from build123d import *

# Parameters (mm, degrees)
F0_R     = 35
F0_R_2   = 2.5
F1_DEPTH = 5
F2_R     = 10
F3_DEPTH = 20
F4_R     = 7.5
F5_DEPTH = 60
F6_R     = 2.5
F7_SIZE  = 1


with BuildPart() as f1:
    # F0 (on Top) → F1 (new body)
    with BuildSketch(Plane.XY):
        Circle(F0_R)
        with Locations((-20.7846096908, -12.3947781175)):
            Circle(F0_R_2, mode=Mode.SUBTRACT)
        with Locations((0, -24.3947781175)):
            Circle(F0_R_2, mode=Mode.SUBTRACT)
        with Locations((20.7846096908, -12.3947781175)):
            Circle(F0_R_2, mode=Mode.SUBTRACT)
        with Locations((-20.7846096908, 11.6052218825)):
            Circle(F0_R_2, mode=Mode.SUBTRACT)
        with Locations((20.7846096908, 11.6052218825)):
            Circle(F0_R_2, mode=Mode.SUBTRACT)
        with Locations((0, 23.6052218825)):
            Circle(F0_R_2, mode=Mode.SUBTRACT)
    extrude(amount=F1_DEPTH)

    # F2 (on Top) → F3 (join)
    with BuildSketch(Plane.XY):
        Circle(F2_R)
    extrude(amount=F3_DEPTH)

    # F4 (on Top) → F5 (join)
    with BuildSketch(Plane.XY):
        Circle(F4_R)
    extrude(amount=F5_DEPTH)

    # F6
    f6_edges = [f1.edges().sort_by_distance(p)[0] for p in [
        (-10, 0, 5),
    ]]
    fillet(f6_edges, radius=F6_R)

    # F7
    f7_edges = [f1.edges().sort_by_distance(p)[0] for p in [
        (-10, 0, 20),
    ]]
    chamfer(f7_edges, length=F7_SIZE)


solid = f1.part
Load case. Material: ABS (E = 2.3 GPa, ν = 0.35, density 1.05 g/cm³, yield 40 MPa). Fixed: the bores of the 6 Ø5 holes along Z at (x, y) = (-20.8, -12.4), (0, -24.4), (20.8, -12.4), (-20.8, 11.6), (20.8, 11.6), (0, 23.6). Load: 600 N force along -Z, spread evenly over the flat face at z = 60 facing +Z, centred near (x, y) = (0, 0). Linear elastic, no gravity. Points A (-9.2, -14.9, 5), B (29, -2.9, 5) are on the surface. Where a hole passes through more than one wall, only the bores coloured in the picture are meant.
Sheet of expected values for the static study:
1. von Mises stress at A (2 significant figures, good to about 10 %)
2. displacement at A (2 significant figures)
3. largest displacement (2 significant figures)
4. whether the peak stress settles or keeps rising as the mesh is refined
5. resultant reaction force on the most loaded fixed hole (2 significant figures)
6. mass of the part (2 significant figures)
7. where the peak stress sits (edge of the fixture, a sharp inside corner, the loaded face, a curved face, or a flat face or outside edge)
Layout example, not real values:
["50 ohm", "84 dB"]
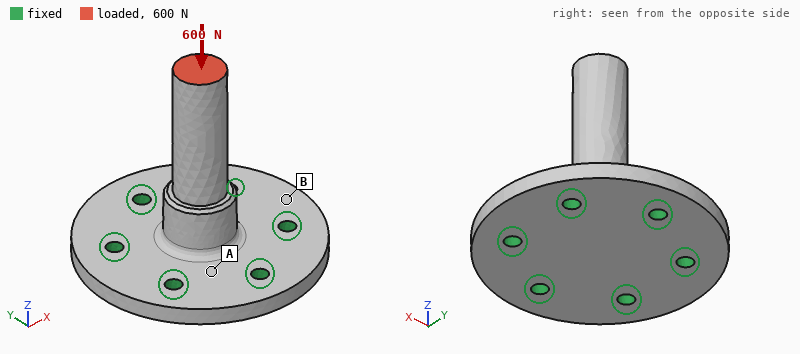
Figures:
["2.8 MPa", "0.040 mm", "0.16 mm", "keeps rising", "110 N", "32 g", "edge of the fixture"]
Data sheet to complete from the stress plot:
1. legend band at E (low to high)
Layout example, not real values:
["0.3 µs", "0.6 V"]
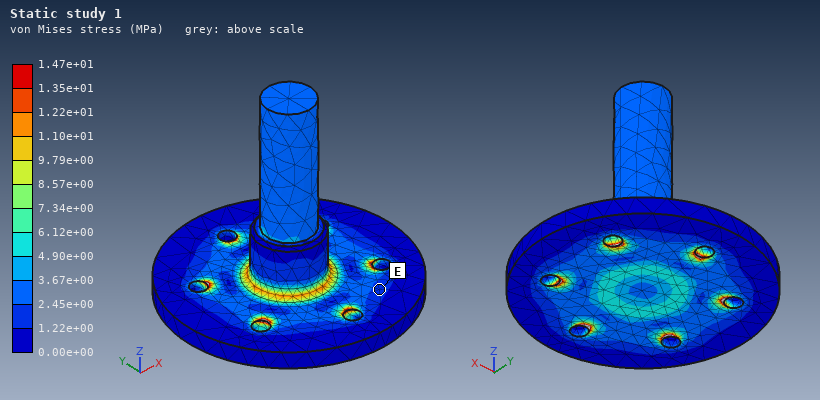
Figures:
["1.22e+00 to 2.45e+00 MPa"]
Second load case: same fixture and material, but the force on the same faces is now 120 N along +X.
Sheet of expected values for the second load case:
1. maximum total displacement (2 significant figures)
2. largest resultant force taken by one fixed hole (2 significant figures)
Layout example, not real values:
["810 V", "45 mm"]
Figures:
["1.1 mm", "110 N"]
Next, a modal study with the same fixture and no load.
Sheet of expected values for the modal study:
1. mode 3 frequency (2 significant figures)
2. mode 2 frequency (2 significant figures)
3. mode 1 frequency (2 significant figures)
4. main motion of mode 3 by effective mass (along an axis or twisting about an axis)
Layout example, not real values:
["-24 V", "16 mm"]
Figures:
["3100 Hz", "1000 Hz", "1000 Hz", "along Z"]
